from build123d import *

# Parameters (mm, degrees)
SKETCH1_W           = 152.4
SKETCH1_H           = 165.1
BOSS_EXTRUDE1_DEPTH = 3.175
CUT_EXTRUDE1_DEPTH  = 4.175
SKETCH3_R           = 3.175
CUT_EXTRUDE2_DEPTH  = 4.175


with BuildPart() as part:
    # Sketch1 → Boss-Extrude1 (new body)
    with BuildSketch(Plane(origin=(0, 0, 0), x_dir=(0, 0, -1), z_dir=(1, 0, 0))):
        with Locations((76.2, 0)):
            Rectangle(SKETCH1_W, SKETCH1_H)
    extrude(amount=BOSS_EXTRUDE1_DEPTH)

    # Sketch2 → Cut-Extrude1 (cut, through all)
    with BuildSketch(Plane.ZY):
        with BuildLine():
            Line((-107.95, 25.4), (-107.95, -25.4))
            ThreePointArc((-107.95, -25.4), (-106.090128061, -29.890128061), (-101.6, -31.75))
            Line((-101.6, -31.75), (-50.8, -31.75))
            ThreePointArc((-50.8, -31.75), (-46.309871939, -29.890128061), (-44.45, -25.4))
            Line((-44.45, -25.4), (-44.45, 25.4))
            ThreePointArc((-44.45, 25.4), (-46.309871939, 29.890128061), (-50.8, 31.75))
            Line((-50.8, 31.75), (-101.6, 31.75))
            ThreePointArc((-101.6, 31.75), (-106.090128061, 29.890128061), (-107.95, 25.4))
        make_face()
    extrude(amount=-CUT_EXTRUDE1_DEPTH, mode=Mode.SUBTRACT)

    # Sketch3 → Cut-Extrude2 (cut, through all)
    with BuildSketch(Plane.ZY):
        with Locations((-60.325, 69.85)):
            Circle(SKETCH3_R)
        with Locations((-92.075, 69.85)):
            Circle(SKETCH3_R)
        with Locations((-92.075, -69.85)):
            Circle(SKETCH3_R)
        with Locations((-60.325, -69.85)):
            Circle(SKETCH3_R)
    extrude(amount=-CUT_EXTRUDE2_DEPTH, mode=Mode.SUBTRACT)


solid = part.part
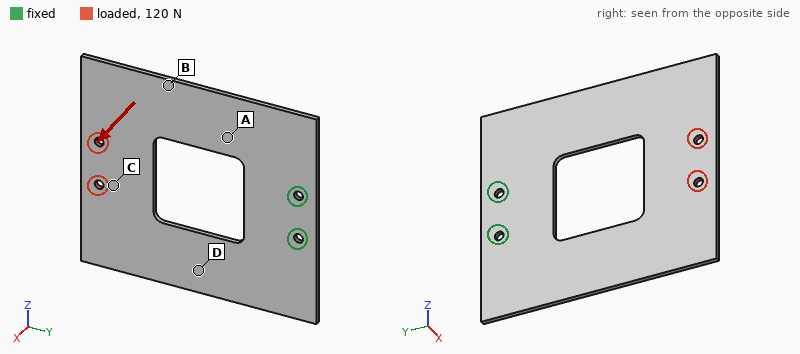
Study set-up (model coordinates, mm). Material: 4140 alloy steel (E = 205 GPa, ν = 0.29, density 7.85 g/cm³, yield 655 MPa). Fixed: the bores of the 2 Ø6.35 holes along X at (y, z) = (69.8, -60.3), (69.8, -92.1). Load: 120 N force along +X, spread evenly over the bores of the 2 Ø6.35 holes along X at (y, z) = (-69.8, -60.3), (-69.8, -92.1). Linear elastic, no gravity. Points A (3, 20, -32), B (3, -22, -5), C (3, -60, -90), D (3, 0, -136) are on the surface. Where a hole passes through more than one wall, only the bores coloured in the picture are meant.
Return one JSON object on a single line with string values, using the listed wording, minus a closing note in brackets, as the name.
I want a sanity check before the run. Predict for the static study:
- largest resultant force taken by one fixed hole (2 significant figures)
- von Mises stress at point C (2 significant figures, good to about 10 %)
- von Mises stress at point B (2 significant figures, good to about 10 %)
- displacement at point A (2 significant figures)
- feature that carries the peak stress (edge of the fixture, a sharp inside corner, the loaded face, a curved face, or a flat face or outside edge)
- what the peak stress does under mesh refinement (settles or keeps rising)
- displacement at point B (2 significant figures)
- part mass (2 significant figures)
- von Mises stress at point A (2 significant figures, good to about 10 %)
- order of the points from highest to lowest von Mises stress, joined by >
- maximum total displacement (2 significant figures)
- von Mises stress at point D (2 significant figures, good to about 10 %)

{"largest resultant force taken by one fixed hole": "60 N", "von Mises stress at point C": "16 MPa", "von Mises stress at point B": "39 MPa", "displacement at point A": "0.39 mm", "feature that carries the peak stress": "edge of the fixture", "what the peak stress does under mesh refinement": "keeps rising", "displacement at point B": "1.1 mm", "part mass": "520 g", "von Mises stress at point A": "81 MPa", "order of the points from highest to lowest von Mises stress, joined by >": "A > D > B > C", "maximum total displacement": "2.6 mm", "von Mises stress at point D": "57 MPa"}
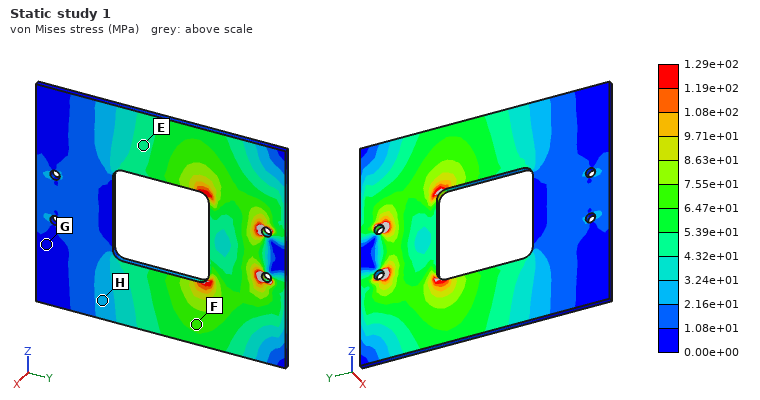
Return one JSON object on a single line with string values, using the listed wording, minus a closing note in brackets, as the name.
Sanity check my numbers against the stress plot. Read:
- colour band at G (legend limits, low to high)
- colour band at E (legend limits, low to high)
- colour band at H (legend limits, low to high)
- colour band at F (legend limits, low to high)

{"colour band at G": "0.00e+00 to 1.08e+01 MPa", "colour band at E": "4.32e+01 to 5.39e+01 MPa", "colour band at H": "2.16e+01 to 3.24e+01 MPa", "colour band at F": "6.47e+01 to 7.55e+01 MPa"}
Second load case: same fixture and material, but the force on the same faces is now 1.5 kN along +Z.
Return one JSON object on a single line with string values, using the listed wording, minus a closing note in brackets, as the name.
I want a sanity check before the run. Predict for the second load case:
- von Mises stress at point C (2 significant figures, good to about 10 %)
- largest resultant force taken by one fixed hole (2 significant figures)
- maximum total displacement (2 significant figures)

{"von Mises stress at point C": "20 MPa", "largest resultant force taken by one fixed hole": "5.6 kN", "maximum total displacement": "0.15 mm"}
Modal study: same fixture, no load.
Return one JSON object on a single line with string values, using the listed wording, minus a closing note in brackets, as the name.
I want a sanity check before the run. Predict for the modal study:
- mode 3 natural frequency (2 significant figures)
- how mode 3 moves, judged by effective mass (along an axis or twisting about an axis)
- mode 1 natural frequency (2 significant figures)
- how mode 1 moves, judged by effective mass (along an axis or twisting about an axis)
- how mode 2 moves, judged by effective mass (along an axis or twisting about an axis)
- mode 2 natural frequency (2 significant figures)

{"mode 3 natural frequency": "480 Hz", "how mode 3 moves, judged by effective mass": "along X", "mode 1 natural frequency": "90 Hz", "how mode 1 moves, judged by effective mass": "along X", "how mode 2 moves, judged by effective mass": "twisting about Y", "mode 2 natural frequency": "190 Hz"}
